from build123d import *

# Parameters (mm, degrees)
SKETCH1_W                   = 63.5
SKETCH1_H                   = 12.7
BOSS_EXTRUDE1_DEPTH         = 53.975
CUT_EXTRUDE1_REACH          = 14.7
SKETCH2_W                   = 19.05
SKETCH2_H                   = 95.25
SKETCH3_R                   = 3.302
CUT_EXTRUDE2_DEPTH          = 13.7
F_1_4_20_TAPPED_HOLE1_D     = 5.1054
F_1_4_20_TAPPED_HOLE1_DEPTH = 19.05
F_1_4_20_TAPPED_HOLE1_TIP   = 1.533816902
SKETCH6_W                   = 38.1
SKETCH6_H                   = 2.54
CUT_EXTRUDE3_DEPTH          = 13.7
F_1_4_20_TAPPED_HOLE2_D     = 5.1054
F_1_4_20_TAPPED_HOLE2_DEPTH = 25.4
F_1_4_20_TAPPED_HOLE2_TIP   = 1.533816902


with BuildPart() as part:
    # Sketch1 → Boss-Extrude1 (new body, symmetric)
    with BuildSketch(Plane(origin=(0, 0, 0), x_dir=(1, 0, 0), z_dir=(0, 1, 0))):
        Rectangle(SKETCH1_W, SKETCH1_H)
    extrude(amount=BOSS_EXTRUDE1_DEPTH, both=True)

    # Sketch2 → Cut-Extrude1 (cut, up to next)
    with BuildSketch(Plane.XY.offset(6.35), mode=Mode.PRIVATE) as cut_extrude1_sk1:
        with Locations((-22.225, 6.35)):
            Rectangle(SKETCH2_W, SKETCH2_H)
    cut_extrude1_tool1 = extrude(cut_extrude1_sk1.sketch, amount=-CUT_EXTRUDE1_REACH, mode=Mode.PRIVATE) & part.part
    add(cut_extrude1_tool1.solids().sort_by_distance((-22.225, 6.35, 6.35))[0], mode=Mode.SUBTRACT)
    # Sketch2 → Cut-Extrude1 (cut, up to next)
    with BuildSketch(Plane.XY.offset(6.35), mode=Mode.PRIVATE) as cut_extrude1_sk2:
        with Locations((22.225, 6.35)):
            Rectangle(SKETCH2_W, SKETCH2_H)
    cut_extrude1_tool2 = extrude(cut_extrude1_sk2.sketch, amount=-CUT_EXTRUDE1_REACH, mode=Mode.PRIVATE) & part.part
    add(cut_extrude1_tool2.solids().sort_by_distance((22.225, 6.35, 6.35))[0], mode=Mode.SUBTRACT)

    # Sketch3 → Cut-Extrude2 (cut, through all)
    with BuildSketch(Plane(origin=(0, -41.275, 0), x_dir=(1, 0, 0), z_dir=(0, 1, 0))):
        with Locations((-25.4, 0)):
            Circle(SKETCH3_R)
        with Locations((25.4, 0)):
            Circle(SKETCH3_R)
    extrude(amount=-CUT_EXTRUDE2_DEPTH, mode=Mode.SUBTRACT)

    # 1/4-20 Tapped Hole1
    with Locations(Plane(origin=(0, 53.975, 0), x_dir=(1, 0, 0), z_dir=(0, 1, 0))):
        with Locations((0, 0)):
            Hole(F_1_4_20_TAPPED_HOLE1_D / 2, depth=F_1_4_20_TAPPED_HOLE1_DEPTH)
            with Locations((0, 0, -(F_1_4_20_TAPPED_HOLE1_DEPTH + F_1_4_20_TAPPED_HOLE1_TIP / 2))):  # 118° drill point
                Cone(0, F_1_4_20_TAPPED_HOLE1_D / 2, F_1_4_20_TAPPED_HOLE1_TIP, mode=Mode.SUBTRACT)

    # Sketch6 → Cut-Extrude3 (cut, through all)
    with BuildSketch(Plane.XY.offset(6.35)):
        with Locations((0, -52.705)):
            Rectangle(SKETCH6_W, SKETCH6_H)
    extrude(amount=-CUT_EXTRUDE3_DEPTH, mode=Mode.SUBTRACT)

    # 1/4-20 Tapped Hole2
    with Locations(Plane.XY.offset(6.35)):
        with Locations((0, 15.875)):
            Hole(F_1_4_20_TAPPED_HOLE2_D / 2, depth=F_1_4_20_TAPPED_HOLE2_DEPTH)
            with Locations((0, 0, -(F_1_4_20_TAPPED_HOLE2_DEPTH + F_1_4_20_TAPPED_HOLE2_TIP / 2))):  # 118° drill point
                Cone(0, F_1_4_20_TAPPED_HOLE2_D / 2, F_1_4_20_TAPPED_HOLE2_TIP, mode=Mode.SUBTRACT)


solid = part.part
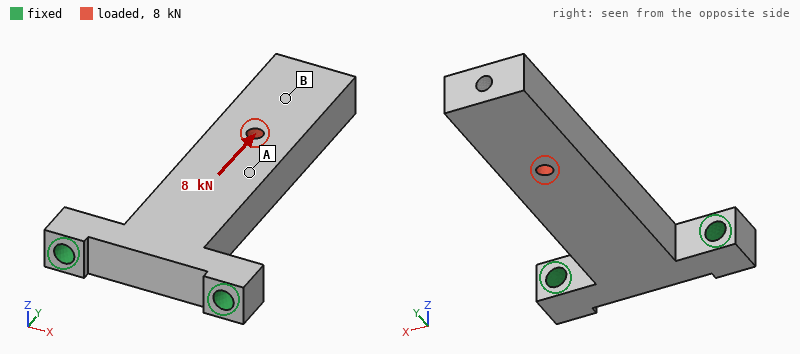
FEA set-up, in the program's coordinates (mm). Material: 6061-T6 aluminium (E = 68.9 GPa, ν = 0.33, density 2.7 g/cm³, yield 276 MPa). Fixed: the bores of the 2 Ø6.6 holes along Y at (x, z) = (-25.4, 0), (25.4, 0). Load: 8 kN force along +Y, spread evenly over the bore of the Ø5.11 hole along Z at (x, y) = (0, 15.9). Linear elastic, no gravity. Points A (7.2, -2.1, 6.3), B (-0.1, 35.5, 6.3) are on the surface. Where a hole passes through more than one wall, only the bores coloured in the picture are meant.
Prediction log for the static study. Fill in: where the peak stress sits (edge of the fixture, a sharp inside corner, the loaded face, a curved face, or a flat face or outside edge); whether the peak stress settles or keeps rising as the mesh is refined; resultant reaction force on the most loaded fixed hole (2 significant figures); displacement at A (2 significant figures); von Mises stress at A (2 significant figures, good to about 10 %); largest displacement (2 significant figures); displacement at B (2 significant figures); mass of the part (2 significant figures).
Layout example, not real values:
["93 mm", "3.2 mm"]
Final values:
["edge of the fixture", "keeps rising", "4.3 kN", "43 µm", "25 MPa", "53 µm", "50 µm", "100 g"]
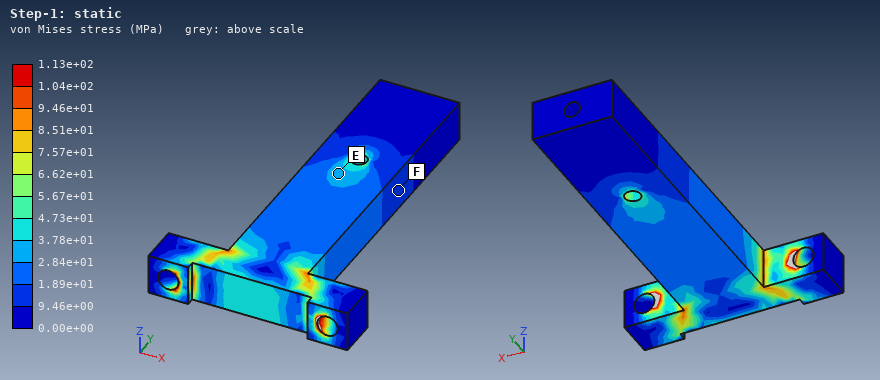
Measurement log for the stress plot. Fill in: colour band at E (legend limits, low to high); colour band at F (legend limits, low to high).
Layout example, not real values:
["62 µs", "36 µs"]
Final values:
["2.84e+01 to 3.78e+01 MPa", "9.46e+00 to 1.89e+01 MPa"]
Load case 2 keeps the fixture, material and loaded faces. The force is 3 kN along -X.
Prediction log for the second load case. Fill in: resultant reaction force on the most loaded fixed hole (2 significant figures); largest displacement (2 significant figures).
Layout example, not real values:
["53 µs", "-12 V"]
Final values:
["5.5 kN", "0.57 mm"]
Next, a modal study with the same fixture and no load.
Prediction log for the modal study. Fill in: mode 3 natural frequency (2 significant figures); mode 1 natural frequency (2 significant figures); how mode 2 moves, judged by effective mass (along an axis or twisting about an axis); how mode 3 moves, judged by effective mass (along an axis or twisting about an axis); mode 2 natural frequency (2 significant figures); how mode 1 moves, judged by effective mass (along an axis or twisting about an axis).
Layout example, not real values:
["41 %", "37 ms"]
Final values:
["4800 Hz", "720 Hz", "along X", "along Z", "1700 Hz", "along Z"]
